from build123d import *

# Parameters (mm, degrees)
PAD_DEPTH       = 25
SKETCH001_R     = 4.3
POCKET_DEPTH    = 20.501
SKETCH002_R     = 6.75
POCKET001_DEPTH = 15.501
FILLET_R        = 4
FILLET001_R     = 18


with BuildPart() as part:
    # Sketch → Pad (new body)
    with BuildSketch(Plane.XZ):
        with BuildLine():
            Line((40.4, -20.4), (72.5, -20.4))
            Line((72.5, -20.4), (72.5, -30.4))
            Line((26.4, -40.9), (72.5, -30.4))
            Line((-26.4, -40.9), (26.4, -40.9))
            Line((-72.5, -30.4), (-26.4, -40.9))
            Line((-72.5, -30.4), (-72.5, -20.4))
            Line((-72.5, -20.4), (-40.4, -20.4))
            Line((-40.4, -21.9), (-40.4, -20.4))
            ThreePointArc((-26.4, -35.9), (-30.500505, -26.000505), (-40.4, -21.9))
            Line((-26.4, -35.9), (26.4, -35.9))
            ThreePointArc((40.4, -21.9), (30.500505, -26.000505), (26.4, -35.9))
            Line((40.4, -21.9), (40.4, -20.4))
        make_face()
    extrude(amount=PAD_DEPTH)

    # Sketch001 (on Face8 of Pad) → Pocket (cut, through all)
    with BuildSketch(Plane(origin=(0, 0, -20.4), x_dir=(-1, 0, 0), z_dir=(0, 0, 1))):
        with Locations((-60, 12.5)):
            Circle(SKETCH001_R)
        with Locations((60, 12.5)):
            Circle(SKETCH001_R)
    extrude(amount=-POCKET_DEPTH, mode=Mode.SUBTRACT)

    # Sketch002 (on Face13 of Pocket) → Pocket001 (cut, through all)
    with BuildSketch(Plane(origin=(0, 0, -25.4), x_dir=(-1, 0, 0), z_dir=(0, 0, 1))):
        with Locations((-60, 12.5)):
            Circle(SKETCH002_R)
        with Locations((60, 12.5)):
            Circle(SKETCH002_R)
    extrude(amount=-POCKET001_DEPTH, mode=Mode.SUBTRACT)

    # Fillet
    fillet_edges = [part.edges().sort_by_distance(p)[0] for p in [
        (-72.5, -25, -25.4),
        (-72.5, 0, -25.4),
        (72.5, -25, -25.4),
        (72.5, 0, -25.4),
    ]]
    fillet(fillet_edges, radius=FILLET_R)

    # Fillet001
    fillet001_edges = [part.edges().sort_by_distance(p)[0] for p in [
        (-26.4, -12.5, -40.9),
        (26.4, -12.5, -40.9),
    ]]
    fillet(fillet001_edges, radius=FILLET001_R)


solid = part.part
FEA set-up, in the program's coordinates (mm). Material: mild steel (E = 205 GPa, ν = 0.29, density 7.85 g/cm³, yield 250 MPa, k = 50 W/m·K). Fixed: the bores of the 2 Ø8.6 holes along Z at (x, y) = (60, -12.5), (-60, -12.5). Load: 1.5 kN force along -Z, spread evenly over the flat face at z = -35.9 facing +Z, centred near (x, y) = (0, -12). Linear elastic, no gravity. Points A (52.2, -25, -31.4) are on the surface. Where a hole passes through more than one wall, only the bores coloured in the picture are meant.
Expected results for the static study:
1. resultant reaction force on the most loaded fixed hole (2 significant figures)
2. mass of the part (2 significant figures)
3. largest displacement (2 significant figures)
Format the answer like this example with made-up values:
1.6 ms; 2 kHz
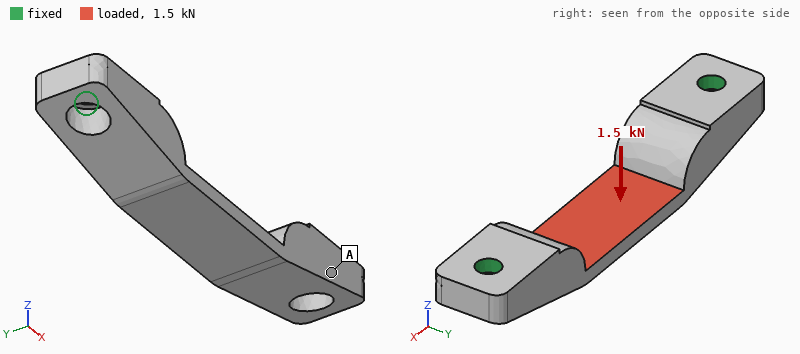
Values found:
1.8 kN; 280 g; 25 µm
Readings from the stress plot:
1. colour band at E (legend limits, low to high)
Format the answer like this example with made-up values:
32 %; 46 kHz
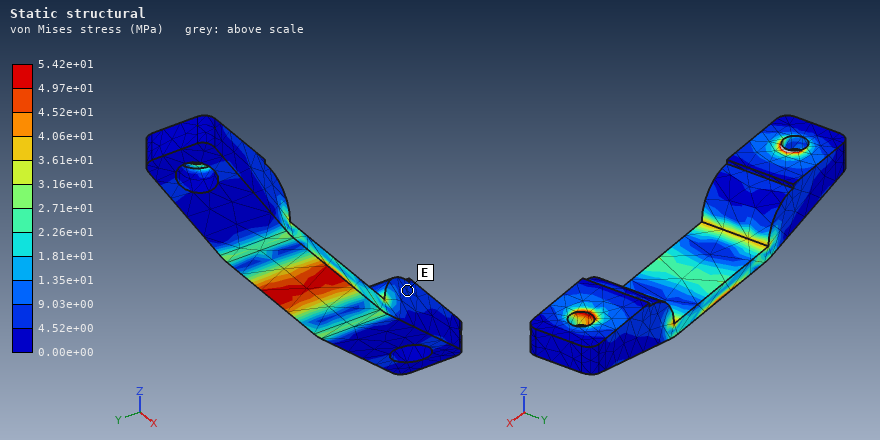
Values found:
4.52e+00 to 9.03e+00 MPa
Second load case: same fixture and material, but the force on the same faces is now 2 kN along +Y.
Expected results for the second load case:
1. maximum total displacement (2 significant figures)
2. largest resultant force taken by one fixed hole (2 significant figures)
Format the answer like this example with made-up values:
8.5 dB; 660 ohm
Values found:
23 µm; 1.0 kN
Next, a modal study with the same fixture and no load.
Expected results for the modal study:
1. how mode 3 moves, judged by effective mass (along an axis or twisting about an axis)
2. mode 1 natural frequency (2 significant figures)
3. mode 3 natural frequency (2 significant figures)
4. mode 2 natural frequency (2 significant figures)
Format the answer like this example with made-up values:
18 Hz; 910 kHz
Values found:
along Z; 4900 Hz; 5800 Hz; 4900 Hz
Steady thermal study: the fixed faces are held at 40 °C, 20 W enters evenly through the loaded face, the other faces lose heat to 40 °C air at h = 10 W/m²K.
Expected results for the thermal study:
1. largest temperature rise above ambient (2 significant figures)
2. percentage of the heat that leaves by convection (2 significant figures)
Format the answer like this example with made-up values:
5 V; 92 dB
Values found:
47 K; 7.9 %
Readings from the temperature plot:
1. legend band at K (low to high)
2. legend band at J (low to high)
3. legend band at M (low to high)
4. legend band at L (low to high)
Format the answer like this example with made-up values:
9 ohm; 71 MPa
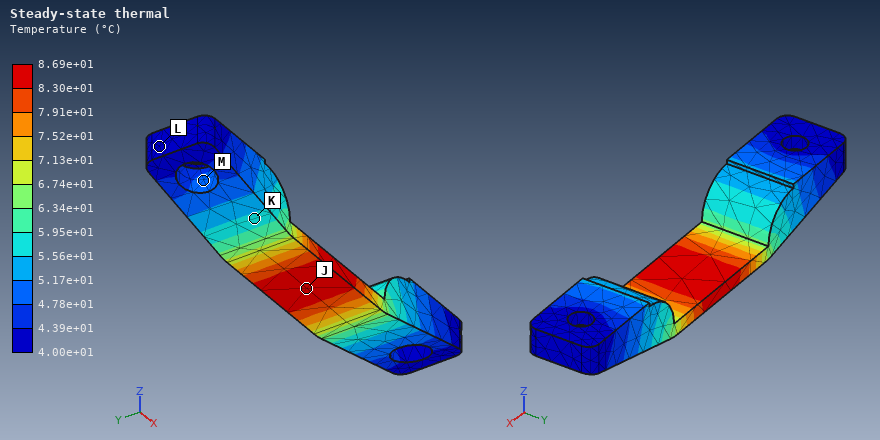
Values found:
5.56e+01 to 5.95e+01 °C; 8.30e+01 to 8.69e+01 °C; 4.78e+01 to 5.17e+01 °C; 4.00e+01 to 4.39e+01 °C
